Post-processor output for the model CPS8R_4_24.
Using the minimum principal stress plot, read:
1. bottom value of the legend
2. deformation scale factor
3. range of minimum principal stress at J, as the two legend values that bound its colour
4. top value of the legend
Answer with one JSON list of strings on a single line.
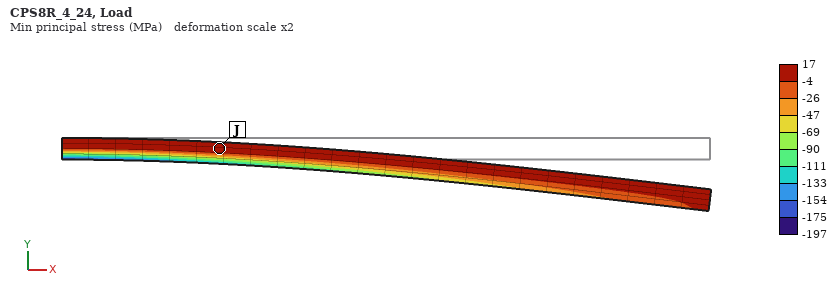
["-197 MPa", "2", "-4 to 17 MPa", "17 MPa"]
